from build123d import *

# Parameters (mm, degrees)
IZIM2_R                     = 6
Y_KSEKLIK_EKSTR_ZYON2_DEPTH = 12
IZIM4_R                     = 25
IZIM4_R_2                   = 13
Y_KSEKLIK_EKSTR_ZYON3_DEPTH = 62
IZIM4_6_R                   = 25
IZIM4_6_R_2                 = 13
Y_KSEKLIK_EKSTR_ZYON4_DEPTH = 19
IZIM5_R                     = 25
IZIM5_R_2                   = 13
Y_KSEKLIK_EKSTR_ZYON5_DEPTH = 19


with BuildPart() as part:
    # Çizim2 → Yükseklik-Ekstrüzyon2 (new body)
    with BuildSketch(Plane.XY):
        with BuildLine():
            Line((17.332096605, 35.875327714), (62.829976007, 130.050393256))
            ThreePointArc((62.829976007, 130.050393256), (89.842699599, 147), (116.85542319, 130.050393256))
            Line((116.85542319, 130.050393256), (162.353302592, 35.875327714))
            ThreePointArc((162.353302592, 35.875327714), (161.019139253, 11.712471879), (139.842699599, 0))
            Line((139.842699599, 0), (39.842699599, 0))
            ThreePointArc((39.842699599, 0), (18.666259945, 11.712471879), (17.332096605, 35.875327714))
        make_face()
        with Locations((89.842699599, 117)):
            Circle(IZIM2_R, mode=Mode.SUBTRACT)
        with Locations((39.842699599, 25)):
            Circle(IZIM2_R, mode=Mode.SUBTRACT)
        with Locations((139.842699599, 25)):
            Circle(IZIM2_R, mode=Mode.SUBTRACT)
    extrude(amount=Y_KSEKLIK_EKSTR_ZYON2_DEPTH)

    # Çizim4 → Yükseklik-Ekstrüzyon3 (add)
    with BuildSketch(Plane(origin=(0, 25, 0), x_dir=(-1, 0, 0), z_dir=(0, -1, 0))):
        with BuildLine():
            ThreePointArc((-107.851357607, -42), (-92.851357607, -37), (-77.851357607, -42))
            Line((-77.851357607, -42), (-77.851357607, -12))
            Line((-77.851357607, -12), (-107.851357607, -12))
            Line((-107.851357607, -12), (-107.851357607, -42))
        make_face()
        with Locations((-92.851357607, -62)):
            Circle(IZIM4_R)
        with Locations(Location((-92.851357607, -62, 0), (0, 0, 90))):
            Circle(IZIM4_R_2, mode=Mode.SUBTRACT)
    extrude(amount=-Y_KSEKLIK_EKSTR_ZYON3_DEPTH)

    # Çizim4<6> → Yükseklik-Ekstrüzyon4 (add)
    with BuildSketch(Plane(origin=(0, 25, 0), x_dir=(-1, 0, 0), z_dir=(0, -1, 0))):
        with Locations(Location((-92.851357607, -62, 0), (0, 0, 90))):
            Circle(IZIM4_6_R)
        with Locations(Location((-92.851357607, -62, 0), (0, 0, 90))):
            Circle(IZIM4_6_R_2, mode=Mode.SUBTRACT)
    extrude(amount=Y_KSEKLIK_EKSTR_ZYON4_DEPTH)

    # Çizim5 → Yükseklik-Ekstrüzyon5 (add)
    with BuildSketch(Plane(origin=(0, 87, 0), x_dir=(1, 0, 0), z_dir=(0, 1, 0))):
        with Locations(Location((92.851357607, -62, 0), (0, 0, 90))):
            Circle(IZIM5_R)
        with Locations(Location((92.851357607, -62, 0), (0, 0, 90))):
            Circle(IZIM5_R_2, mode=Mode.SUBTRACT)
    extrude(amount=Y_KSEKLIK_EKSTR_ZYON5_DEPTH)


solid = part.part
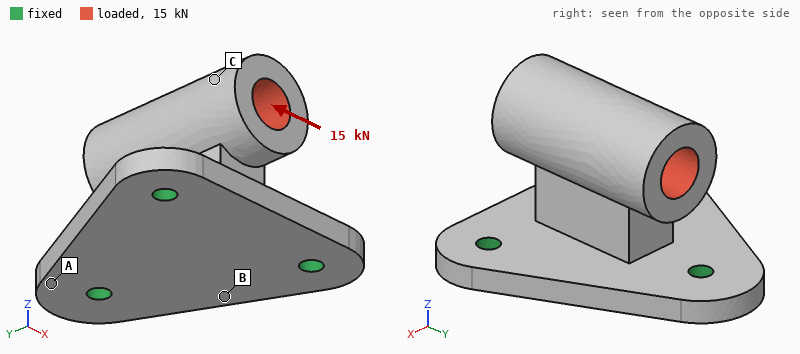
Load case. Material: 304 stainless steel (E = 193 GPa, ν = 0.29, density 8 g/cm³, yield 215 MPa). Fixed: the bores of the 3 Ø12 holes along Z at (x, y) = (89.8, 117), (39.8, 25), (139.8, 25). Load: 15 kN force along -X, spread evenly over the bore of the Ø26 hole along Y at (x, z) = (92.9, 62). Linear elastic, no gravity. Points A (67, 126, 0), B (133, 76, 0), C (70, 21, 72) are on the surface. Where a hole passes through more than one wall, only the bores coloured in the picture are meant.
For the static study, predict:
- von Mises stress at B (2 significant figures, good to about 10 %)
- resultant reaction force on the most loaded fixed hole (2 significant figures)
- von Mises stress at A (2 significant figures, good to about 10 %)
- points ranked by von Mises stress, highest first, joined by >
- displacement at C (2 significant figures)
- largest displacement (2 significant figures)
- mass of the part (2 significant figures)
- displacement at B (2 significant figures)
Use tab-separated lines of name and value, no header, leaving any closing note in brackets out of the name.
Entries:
von Mises stress at B	53 MPa
resultant reaction force on the most loaded fixed hole	11 kN
von Mises stress at A	27 MPa
points ranked by von Mises stress, highest first, joined by >	B > A > C
displacement at C	0.15 mm
largest displacement	0.18 mm
mass of the part	3.0 kg
displacement at B	0.036 mm
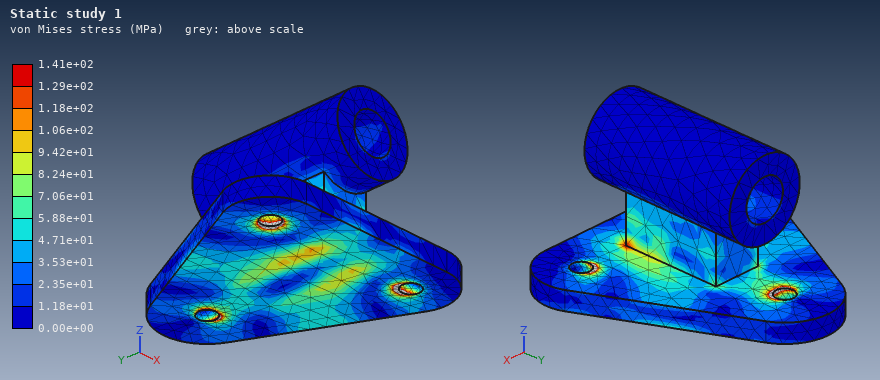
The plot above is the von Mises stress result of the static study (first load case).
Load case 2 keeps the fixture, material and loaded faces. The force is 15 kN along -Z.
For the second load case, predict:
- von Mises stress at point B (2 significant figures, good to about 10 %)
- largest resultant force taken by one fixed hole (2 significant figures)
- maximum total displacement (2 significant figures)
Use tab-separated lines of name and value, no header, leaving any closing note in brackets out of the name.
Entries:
von Mises stress at point B	20 MPa
largest resultant force taken by one fixed hole	5.5 kN
maximum total displacement	28 µm
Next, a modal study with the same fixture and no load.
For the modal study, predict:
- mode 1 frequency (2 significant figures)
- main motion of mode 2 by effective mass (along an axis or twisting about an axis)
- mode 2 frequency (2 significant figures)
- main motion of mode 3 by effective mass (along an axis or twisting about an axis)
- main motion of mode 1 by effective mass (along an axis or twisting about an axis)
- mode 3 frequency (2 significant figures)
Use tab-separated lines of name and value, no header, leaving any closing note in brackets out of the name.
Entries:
mode 1 frequency	1500 Hz
main motion of mode 2 by effective mass	along Y
mode 2 frequency	1900 Hz
main motion of mode 3 by effective mass	along Z
main motion of mode 1 by effective mass	along X
mode 3 frequency	2900 Hz
